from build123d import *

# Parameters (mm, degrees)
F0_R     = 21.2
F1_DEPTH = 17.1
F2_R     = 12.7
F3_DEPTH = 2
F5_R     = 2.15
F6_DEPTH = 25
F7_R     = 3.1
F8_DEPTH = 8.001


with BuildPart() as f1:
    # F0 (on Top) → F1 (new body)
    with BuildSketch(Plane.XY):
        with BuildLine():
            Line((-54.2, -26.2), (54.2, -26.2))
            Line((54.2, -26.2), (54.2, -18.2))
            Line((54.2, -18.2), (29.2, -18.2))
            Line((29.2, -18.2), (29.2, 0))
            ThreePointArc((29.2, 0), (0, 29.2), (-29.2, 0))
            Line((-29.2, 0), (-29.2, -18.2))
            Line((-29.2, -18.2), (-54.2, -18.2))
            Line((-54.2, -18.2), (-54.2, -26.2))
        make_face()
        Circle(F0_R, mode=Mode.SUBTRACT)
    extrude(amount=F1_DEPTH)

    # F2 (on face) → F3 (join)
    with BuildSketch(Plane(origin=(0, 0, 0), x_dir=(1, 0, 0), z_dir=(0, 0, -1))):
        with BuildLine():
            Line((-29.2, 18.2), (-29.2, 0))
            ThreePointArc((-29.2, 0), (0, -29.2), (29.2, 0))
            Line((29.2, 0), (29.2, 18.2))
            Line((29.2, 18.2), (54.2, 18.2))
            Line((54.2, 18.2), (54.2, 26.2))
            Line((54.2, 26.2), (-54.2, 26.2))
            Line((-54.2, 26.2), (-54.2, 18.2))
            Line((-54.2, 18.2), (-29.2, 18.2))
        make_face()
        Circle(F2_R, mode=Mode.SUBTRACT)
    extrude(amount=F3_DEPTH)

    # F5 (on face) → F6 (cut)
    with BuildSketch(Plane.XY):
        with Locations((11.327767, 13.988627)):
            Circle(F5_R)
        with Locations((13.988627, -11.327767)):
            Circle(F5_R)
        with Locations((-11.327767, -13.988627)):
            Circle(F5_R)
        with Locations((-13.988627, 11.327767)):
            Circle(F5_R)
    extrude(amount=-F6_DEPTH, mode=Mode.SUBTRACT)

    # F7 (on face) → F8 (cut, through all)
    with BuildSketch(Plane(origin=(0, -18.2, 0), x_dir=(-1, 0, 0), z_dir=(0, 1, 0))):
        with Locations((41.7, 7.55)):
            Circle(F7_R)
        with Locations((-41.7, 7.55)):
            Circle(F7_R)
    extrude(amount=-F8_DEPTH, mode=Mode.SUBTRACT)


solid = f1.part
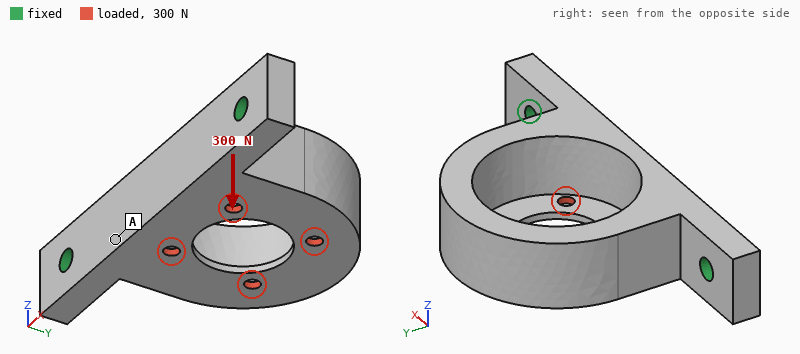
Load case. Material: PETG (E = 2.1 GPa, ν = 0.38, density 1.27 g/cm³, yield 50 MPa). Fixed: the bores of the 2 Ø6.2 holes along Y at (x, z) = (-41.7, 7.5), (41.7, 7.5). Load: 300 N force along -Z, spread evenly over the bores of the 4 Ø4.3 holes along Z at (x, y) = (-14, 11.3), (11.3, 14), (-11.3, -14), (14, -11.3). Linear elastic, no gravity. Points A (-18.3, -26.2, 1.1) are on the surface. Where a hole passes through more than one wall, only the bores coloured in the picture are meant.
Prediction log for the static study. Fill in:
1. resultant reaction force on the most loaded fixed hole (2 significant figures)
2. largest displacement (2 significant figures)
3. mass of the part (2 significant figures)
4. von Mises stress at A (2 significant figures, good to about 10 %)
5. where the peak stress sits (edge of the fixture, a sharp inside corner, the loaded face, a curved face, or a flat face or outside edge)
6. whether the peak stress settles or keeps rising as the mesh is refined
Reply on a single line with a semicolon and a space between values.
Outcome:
150 N; 1.3 mm; 47 g; 2.9 MPa; edge of the fixture; keeps rising
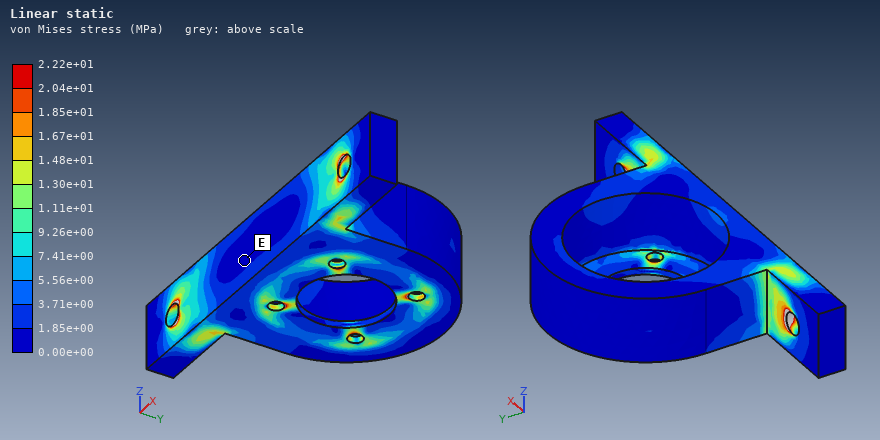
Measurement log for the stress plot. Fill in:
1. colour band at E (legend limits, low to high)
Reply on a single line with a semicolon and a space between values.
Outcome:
0.00e+00 to 1.85e+00 MPa
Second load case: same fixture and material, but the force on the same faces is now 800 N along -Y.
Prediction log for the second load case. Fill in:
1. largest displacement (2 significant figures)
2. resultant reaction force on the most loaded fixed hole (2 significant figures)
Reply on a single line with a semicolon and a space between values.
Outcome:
1.4 mm; 420 N
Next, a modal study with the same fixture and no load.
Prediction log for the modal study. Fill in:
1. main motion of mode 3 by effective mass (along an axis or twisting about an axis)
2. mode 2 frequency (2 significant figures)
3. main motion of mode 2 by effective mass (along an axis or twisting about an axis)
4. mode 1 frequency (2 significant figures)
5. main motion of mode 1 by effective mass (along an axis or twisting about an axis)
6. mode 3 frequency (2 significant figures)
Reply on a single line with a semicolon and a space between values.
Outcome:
along Y; 1300 Hz; along X; 490 Hz; along Z; 1600 Hz
